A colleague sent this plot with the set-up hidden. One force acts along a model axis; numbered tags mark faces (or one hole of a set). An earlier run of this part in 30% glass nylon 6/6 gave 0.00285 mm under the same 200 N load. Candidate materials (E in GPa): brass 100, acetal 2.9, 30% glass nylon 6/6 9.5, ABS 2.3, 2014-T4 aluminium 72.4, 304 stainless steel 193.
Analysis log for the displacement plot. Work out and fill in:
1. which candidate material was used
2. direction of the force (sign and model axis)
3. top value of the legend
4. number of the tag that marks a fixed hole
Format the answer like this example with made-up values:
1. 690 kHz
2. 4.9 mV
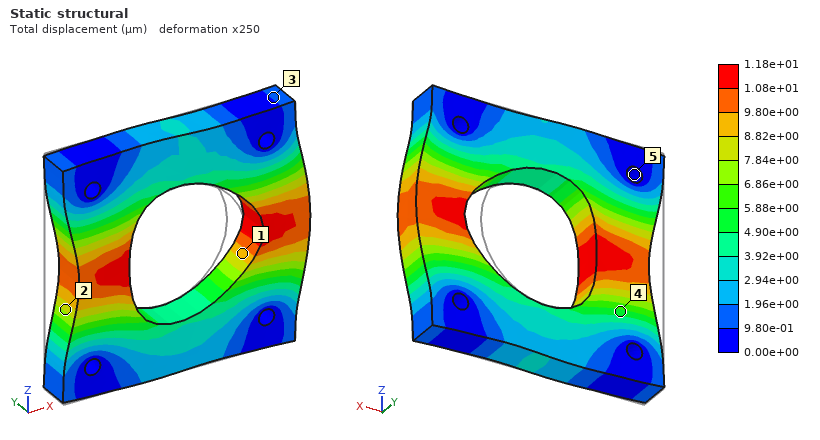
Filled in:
1. ABS
2. +X
3. 1.18e+01 µm
4. 5
